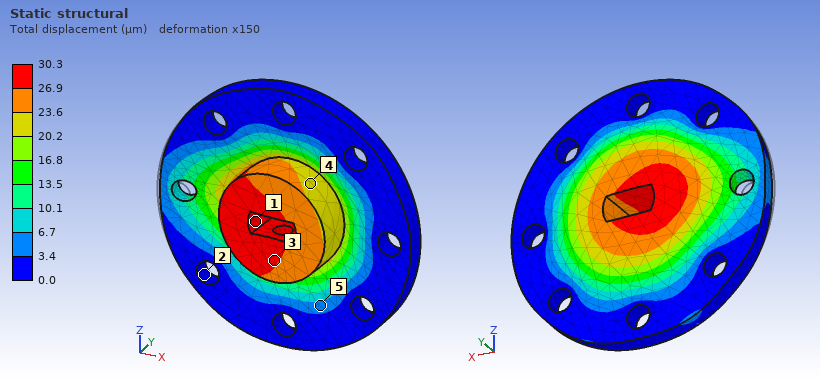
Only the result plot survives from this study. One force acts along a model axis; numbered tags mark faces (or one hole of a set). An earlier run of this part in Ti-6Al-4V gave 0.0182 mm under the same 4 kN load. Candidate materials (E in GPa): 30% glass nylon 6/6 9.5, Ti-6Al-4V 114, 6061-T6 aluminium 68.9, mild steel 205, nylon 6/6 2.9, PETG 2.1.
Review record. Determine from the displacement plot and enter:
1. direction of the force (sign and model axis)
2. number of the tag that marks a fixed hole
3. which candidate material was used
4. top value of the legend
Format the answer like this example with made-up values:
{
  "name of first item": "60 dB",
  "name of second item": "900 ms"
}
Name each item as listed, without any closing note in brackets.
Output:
{
  "direction of the force": "+Y",
  "number of the tag that marks a fixed hole": "2",
  "which candidate material was used": "6061-T6 aluminium",
  "top value of the legend": "30.3 µm"
}
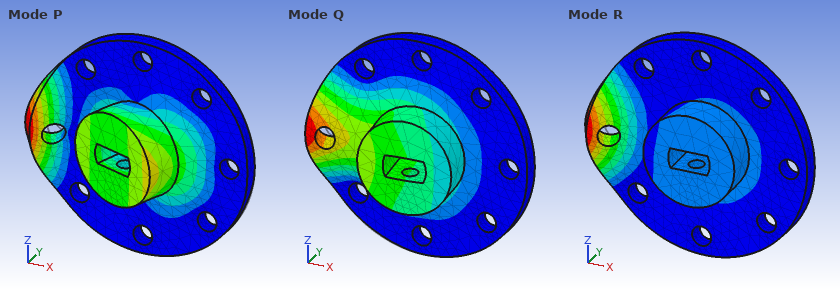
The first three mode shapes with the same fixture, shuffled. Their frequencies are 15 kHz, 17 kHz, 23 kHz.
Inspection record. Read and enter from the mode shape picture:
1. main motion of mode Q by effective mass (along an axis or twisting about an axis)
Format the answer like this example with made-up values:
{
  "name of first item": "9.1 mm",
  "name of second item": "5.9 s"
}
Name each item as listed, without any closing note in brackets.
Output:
{
  "main motion of mode Q by effective mass": "along Y"
}
